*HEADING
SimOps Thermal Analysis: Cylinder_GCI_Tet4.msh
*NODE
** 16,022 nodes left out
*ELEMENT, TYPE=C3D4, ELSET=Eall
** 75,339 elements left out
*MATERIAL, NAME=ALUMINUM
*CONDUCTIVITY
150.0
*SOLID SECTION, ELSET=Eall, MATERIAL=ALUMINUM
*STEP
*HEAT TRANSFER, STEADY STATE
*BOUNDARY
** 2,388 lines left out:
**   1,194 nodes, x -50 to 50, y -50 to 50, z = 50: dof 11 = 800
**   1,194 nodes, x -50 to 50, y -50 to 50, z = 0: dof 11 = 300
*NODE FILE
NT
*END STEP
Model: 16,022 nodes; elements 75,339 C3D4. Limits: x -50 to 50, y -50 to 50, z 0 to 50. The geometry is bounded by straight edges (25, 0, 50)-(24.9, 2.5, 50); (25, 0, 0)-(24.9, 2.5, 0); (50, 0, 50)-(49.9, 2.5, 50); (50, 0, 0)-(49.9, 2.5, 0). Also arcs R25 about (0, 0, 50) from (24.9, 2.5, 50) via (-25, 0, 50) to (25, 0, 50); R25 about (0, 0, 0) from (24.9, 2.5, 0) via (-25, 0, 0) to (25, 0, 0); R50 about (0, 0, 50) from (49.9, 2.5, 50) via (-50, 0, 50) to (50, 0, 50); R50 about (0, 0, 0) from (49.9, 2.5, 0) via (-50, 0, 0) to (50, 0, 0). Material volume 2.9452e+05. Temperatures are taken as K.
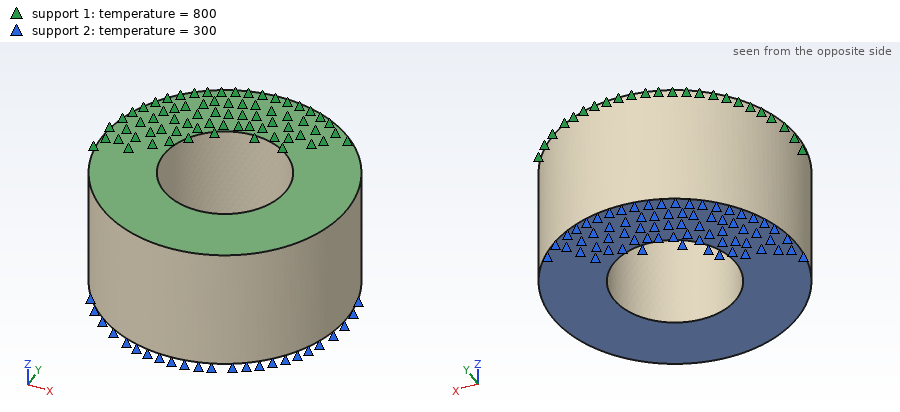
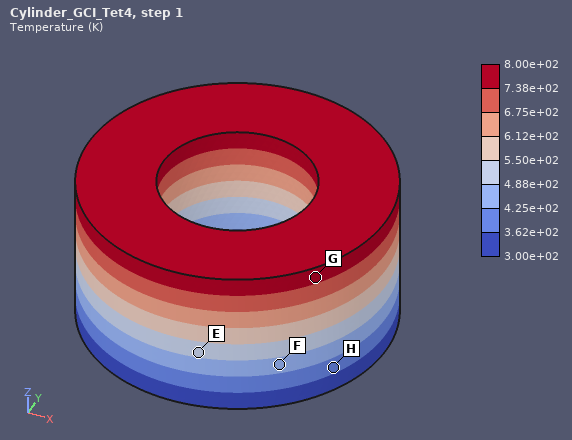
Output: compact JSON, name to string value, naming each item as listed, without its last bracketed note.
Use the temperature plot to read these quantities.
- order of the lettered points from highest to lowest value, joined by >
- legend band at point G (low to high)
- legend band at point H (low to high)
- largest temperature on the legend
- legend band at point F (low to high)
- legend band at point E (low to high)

{"order of the lettered points from highest to lowest value, joined by >": "G > E > F > H", "legend band at point G": "7.38e+02 to 8.00e+02 K", "legend band at point H": "3.62e+02 to 4.25e+02 K", "largest temperature on the legend": "8.00e+02 K", "legend band at point F": "4.25e+02 to 4.88e+02 K", "legend band at point E": "4.88e+02 to 5.50e+02 K"}
